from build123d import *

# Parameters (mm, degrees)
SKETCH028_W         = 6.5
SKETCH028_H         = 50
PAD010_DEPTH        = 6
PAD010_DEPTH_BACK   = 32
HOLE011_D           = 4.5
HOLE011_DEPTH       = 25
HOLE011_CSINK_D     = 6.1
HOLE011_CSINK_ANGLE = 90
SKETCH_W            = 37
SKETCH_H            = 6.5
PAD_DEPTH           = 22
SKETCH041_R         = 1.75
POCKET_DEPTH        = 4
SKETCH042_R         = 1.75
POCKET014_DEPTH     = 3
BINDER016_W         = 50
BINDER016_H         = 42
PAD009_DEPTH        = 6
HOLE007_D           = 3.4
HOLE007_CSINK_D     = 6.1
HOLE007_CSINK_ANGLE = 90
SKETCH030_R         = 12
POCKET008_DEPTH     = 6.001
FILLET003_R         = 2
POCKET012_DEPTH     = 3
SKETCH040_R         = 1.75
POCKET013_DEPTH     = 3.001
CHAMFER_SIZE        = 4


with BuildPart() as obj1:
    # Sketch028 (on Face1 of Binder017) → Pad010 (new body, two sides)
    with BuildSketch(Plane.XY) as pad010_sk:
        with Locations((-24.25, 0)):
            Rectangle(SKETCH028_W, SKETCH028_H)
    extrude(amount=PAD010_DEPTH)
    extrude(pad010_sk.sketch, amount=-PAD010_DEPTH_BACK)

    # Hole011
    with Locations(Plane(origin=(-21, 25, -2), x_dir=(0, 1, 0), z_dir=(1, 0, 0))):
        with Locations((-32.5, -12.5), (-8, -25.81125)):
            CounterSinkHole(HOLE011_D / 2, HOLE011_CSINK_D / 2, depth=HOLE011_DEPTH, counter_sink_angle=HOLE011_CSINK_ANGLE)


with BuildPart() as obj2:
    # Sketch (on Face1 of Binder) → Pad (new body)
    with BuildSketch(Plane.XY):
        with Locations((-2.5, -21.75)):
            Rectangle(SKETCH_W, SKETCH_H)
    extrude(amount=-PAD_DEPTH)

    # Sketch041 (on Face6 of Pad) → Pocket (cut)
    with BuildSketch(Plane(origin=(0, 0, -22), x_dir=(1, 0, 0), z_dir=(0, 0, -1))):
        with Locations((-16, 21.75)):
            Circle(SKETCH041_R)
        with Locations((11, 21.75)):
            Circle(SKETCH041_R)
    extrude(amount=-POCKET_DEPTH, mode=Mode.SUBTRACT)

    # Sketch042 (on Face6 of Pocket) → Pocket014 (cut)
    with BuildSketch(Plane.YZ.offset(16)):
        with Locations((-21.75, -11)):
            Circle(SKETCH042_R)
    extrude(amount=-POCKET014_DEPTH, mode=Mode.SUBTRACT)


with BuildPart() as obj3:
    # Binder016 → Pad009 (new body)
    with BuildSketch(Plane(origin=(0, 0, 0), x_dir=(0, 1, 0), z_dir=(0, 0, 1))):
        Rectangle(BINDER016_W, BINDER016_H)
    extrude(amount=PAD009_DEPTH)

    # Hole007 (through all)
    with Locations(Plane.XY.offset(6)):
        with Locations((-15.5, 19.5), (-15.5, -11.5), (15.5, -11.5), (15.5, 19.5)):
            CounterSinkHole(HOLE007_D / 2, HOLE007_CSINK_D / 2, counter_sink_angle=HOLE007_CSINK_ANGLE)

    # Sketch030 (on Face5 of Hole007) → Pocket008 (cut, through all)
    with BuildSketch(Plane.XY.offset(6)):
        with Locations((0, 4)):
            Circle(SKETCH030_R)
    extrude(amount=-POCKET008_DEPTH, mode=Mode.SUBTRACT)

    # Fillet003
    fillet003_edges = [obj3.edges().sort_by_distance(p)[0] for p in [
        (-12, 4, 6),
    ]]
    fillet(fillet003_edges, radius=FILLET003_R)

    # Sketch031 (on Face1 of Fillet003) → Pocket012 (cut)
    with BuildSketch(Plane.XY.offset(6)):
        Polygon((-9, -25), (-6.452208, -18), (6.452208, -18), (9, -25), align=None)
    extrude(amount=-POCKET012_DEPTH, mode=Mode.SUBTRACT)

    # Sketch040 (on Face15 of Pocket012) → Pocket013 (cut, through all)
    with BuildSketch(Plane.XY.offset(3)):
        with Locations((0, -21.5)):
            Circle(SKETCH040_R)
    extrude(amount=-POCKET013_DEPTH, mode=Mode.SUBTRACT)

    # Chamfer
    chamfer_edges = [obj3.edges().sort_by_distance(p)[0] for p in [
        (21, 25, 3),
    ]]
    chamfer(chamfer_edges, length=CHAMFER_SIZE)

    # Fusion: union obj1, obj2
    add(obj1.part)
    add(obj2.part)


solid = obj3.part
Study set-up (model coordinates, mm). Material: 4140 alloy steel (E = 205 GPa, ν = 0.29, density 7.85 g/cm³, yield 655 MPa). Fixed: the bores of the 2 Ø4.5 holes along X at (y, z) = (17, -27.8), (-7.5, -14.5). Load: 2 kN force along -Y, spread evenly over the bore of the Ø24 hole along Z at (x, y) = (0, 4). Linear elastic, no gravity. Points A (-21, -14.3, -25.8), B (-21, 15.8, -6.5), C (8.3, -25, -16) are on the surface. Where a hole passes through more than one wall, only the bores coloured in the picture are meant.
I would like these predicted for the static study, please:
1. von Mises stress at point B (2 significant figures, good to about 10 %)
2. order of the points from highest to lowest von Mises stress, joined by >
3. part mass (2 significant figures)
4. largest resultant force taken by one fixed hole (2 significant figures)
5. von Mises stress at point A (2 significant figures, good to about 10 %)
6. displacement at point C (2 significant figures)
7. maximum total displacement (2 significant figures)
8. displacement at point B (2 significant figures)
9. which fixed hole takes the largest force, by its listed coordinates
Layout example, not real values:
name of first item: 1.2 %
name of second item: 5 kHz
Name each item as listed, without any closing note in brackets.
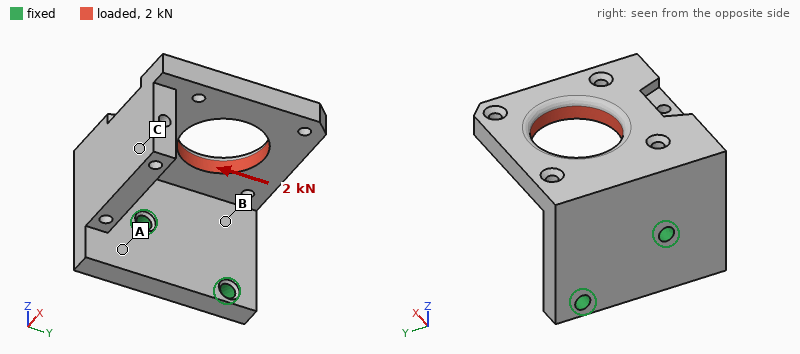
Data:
von Mises stress at point B: 72 MPa
order of the points from highest to lowest von Mises stress, joined by >: B > A > C
part mass: 210 g
largest resultant force taken by one fixed hole: 2.5 kN
von Mises stress at point A: 42 MPa
displacement at point C: 0.070 mm
maximum total displacement: 0.10 mm
displacement at point B: 0.026 mm
which fixed hole takes the largest force, by its listed coordinates: (-7.5, -14.5)
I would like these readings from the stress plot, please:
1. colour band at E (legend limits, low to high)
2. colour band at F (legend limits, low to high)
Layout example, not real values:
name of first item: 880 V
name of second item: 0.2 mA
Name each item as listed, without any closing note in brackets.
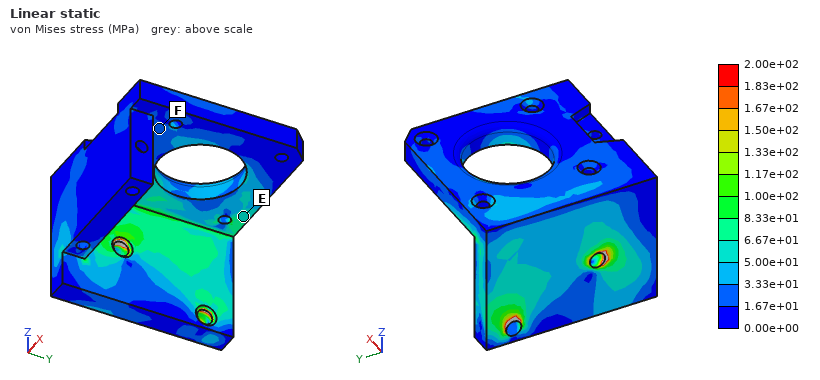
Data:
colour band at E: 5.00e+01 to 6.67e+01 MPa
colour band at F: 1.67e+01 to 3.33e+01 MPa
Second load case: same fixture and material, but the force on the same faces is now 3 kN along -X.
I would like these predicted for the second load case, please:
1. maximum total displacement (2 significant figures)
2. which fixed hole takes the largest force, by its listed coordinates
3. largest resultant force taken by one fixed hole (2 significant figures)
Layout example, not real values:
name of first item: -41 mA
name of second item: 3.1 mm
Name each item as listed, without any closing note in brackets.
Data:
maximum total displacement: 0.13 mm
which fixed hole takes the largest force, by its listed coordinates: (-7.5, -14.5)
largest resultant force taken by one fixed hole: 2.5 kN
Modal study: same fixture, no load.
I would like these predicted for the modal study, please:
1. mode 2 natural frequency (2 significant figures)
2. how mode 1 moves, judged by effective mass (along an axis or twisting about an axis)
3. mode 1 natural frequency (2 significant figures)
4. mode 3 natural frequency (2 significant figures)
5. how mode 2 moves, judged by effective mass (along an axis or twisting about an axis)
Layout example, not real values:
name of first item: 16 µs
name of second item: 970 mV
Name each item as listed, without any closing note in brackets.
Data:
mode 2 natural frequency: 2400 Hz
how mode 1 moves, judged by effective mass: along Z
mode 1 natural frequency: 2000 Hz
mode 3 natural frequency: 4300 Hz
how mode 2 moves, judged by effective mass: along Y
